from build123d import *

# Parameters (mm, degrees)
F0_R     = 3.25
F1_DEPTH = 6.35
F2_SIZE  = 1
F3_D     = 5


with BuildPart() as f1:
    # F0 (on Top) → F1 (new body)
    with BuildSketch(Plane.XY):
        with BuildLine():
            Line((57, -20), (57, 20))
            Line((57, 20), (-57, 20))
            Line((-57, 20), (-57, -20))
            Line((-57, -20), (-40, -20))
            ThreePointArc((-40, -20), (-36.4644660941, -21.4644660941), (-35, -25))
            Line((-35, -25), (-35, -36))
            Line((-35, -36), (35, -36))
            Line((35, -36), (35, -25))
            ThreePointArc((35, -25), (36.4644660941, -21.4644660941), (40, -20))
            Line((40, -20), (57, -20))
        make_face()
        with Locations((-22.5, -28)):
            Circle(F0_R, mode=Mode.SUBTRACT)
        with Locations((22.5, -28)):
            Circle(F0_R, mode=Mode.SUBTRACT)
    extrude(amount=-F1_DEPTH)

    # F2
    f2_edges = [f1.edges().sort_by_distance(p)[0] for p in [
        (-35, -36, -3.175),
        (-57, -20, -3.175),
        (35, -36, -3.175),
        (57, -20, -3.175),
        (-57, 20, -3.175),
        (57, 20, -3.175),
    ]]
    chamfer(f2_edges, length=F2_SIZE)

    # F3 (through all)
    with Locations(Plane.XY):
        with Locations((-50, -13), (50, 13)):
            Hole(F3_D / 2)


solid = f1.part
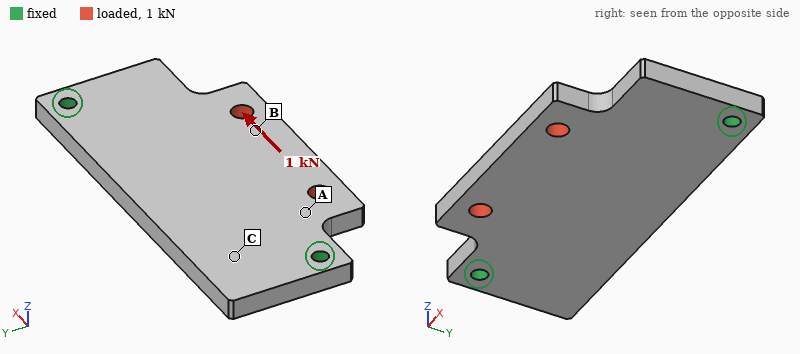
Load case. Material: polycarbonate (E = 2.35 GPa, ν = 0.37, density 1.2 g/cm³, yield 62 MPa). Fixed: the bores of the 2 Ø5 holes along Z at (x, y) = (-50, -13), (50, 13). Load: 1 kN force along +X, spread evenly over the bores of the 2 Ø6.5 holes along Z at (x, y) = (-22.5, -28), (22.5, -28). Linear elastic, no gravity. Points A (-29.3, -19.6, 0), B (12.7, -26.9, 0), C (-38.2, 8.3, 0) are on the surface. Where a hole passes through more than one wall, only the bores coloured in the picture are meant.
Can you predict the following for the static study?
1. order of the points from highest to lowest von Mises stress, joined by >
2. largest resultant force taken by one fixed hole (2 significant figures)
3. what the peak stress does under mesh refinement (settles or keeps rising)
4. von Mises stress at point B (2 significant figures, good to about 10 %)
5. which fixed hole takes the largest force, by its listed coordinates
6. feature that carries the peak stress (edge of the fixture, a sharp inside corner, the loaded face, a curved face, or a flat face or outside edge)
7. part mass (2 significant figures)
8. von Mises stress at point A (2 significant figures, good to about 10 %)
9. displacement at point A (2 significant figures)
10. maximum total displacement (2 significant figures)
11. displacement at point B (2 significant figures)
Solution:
A > B > C
650 N
keeps rising
3.4 MPa
(-50, -13)
edge of the fixture
43 g
6.7 MPa
0.072 mm
0.15 mm
0.12 mm
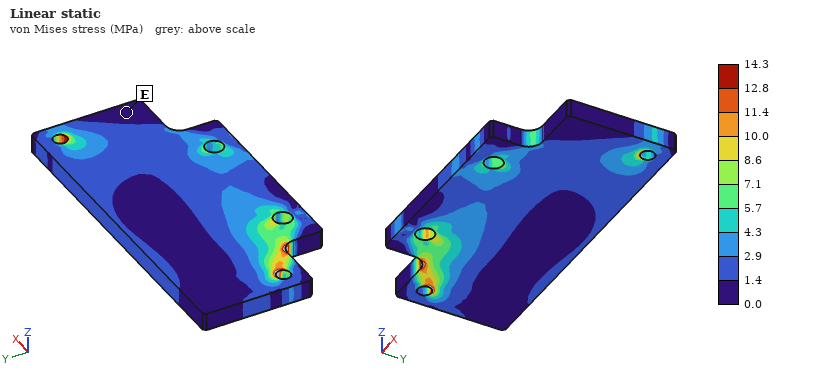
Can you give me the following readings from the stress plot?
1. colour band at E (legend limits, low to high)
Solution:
0.0 to 1.4 MPa
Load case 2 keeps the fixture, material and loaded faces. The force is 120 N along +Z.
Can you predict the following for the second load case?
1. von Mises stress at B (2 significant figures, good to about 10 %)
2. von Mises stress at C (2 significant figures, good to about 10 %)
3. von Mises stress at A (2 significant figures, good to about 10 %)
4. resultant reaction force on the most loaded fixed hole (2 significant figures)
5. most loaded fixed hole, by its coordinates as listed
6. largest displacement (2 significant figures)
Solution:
2.9 MPa
2.3 MPa
5.4 MPa
70 N
(-50, -13)
1.3 mm
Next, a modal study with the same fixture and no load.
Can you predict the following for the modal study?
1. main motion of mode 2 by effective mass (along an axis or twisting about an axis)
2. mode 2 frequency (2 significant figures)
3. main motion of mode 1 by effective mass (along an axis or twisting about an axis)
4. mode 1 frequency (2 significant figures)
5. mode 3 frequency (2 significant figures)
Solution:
along Z
760 Hz
along Z
520 Hz
1400 Hz
